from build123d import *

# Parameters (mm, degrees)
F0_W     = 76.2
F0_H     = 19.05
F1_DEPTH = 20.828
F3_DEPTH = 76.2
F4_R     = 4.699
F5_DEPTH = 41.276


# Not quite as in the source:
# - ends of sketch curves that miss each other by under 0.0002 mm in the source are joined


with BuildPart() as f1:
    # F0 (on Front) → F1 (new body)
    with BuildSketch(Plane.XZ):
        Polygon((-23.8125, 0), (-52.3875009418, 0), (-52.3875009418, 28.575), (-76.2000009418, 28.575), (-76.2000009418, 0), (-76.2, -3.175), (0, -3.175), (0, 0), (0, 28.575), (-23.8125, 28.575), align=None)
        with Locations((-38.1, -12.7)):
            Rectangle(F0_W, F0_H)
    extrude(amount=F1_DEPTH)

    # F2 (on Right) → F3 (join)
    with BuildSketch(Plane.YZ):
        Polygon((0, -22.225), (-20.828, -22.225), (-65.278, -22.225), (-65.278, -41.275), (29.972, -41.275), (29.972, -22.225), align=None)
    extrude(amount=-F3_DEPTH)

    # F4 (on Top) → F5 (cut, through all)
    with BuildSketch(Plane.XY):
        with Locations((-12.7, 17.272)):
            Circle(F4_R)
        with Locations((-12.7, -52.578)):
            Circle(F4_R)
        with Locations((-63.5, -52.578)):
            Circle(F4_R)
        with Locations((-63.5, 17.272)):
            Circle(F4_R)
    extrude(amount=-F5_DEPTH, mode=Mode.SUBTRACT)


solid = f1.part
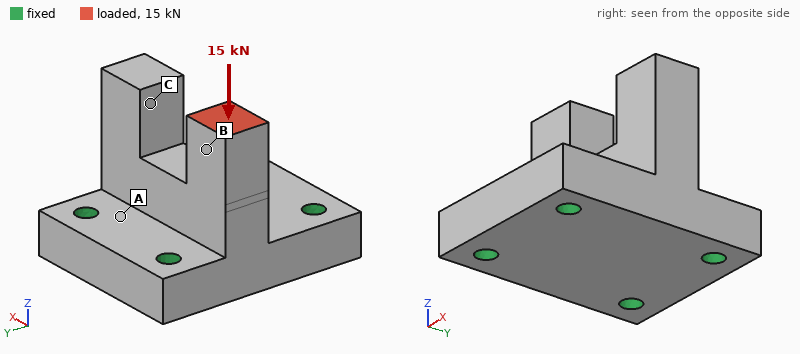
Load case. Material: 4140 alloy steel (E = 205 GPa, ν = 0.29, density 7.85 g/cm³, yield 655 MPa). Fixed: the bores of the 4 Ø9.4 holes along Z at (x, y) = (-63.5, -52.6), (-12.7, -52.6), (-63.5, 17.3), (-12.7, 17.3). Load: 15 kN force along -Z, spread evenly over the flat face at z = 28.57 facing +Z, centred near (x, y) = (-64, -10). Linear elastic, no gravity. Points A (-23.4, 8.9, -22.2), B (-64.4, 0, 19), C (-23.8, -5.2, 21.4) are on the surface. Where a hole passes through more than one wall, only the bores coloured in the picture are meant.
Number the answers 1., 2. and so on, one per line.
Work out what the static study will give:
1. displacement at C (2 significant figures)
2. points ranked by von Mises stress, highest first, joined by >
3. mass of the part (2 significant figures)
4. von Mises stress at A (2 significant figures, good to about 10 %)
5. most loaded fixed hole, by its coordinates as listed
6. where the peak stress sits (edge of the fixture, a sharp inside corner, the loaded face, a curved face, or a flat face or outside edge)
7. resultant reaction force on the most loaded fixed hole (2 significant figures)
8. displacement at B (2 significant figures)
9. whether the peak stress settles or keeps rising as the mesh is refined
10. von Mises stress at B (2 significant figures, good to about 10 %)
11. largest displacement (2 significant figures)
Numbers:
1. 7.4 µm
2. B > A > C
3. 1.5 kg
4. 12 MPa
5. (-63.5, 17.3)
6. edge of the fixture
7. 9.2 kN
8. 18 µm
9. keeps rising
10. 30 MPa
11. 24 µm
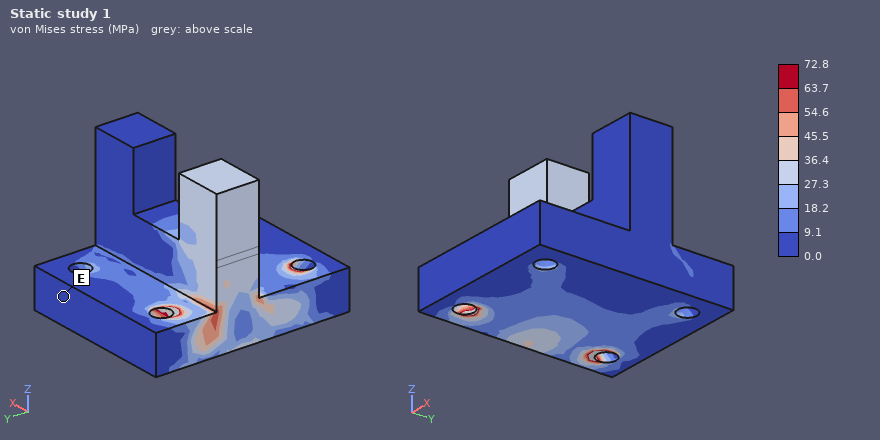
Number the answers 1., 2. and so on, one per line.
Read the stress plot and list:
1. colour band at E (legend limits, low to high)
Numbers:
1. 0.0 to 9.1 MPa
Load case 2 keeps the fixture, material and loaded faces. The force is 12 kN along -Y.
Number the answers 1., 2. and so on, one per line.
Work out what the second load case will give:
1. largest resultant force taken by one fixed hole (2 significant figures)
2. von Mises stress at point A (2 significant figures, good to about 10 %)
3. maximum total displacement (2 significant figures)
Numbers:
1. 11 kN
2. 19 MPa
3. 0.18 mm
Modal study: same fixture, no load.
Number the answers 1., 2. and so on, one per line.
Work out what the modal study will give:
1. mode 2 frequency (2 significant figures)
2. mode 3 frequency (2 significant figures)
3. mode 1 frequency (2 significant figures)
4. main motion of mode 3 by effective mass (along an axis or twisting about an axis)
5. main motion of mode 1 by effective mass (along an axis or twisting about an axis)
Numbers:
1. 5900 Hz
2. 6300 Hz
3. 5100 Hz
4. along X
5. along Y
